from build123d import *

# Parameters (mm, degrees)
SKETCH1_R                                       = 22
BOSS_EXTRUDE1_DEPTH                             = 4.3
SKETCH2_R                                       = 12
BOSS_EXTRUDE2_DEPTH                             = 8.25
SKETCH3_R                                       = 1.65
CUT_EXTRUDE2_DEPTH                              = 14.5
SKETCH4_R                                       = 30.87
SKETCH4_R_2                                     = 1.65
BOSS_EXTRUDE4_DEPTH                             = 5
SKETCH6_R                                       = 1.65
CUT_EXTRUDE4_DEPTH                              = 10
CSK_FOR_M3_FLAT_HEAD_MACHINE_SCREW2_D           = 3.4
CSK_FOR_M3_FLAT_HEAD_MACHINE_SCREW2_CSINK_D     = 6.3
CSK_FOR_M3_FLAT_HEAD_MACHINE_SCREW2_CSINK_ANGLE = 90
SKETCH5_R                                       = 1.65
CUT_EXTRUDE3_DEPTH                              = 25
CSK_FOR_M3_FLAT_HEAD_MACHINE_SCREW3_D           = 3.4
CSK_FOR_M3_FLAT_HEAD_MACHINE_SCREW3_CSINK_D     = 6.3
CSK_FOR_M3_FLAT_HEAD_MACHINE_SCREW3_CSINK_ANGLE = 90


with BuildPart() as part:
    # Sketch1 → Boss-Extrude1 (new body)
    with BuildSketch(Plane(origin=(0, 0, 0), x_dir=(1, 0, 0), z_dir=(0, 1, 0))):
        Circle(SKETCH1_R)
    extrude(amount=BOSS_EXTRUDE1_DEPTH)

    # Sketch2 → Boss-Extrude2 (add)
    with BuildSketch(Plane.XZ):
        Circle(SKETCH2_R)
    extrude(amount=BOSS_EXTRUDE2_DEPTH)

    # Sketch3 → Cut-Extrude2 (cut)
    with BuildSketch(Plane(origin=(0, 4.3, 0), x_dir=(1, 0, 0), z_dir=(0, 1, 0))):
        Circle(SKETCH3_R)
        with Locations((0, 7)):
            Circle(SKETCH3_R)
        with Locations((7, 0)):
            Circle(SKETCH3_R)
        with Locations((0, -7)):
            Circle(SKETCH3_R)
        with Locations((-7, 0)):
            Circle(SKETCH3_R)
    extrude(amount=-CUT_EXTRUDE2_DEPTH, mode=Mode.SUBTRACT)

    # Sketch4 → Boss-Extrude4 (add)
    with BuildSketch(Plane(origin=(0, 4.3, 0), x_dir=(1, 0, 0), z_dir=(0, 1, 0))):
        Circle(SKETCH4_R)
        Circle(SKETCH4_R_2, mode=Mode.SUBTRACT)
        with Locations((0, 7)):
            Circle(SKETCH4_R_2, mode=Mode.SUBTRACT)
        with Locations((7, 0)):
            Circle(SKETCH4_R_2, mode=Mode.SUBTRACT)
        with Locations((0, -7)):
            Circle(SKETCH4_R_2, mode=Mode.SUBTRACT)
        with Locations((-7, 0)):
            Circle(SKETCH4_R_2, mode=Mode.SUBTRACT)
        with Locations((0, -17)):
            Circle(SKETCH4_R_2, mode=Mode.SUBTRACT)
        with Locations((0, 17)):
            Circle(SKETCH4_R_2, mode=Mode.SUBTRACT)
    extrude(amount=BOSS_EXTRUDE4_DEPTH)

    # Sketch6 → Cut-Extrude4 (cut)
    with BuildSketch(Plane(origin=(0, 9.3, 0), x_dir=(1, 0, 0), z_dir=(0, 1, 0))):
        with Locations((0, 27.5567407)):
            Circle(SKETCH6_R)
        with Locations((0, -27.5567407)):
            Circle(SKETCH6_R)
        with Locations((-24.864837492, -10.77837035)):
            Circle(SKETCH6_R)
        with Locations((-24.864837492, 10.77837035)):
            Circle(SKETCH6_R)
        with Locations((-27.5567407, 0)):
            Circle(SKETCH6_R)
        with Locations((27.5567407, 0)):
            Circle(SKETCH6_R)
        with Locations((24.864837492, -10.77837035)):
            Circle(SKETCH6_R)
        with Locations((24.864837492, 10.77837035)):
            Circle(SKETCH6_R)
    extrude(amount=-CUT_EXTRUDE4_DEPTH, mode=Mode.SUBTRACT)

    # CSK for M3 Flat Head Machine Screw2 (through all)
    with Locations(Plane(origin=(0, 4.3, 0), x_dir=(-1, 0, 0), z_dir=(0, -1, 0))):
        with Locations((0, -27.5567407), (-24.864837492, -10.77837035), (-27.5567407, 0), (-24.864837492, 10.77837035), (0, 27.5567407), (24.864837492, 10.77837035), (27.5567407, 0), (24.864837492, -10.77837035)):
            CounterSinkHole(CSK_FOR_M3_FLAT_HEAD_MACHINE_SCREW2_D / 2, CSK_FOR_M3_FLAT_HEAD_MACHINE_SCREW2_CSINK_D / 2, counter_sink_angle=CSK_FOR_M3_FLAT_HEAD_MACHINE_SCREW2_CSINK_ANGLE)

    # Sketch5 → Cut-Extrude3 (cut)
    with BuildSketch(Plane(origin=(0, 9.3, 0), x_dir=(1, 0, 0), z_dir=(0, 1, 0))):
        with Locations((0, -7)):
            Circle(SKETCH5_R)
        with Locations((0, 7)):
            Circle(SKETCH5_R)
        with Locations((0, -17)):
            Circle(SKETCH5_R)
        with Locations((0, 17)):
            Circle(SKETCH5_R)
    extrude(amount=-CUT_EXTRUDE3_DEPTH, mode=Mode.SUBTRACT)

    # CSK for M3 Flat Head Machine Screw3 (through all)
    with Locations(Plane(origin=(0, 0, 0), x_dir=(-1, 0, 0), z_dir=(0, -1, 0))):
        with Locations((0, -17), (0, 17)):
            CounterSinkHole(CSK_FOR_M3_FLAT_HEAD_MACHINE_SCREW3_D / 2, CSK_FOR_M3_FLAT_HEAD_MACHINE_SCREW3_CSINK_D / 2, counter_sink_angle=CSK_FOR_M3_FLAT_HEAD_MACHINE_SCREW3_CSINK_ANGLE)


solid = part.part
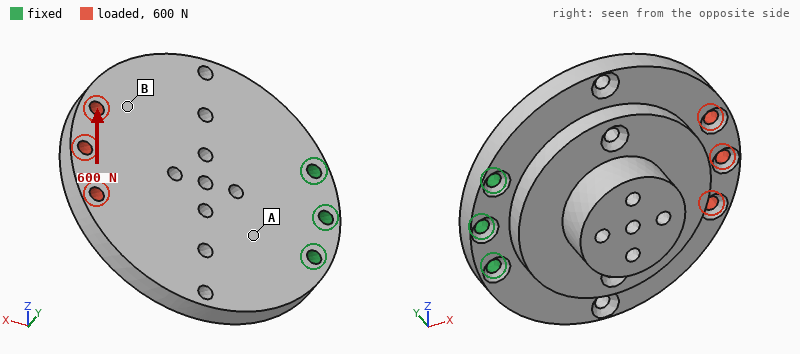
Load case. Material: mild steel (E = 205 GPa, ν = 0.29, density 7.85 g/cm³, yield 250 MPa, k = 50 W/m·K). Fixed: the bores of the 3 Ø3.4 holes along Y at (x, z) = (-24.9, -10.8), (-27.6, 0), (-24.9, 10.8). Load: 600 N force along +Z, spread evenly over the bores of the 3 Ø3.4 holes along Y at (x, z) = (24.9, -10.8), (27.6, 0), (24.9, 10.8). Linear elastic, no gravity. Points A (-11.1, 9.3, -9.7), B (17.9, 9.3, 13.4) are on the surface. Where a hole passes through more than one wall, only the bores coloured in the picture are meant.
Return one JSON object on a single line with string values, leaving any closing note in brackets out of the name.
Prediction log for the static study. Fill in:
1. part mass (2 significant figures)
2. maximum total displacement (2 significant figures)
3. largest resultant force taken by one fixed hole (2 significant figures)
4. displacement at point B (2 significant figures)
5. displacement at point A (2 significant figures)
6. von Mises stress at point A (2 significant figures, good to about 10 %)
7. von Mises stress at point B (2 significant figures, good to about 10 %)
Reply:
{"part mass": "190 g", "maximum total displacement": "11 µm", "largest resultant force taken by one fixed hole": "1.3 kN", "displacement at point B": "8.7 µm", "displacement at point A": "2.8 µm", "von Mises stress at point A": "15 MPa", "von Mises stress at point B": "5.2 MPa"}
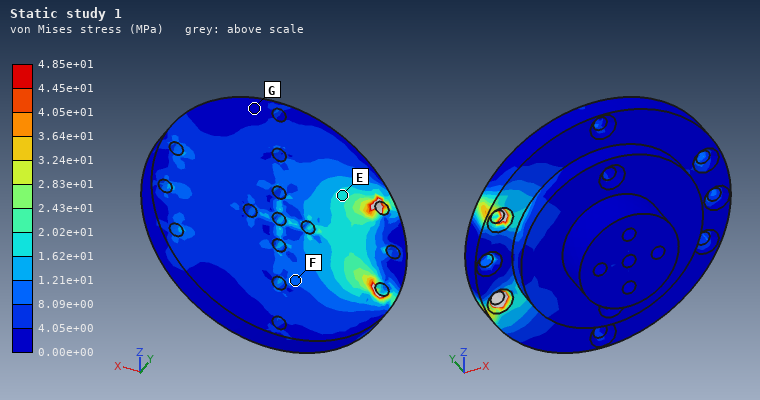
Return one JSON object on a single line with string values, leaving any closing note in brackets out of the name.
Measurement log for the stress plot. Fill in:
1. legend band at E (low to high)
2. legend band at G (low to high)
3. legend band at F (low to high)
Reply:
{"legend band at E": "1.62e+01 to 2.02e+01 MPa", "legend band at G": "0.00e+00 to 4.05e+00 MPa", "legend band at F": "8.09e+00 to 1.21e+01 MPa"}
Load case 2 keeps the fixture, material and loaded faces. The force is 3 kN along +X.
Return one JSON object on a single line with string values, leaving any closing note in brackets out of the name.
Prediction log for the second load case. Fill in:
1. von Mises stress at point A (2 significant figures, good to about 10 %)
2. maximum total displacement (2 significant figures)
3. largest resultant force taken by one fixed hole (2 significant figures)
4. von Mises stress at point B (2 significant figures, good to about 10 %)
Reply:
{"von Mises stress at point A": "24 MPa", "maximum total displacement": "28 µm", "largest resultant force taken by one fixed hole": "1.2 kN", "von Mises stress at point B": "27 MPa"}
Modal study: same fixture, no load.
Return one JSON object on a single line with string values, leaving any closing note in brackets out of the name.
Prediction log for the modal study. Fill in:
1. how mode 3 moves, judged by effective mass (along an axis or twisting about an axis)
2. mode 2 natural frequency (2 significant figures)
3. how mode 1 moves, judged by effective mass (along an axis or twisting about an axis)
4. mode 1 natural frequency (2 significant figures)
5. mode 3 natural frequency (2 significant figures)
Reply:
{"how mode 3 moves, judged by effective mass": "along Z", "mode 2 natural frequency": "4500 Hz", "how mode 1 moves, judged by effective mass": "along Y", "mode 1 natural frequency": "1300 Hz", "mode 3 natural frequency": "5600 Hz"}
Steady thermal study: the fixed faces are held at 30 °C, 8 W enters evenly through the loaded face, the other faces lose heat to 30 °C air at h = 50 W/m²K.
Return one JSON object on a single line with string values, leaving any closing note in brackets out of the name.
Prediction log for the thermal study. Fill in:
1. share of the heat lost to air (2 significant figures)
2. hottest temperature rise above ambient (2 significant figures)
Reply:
{"share of the heat lost to air": "46 %", "hottest temperature rise above ambient": "24 K"}
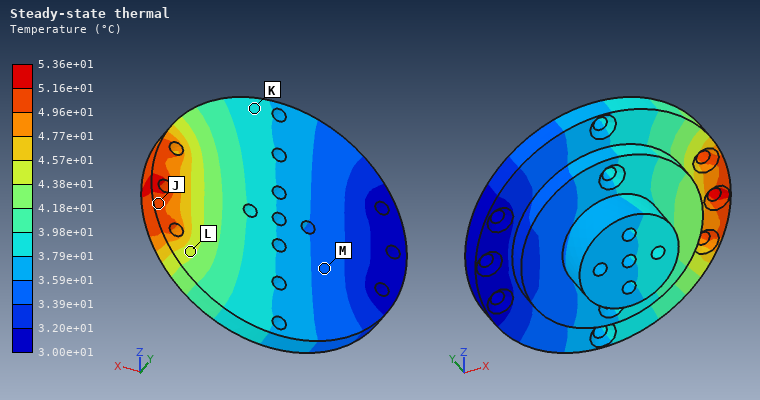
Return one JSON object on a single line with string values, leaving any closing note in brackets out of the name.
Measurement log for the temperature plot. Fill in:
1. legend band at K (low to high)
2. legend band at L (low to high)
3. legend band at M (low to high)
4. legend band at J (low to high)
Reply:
{"legend band at K": "3.79e+01 to 3.98e+01 °C", "legend band at L": "4.38e+01 to 4.57e+01 °C", "legend band at M": "3.39e+01 to 3.59e+01 °C", "legend band at J": "4.96e+01 to 5.16e+01 °C"}
